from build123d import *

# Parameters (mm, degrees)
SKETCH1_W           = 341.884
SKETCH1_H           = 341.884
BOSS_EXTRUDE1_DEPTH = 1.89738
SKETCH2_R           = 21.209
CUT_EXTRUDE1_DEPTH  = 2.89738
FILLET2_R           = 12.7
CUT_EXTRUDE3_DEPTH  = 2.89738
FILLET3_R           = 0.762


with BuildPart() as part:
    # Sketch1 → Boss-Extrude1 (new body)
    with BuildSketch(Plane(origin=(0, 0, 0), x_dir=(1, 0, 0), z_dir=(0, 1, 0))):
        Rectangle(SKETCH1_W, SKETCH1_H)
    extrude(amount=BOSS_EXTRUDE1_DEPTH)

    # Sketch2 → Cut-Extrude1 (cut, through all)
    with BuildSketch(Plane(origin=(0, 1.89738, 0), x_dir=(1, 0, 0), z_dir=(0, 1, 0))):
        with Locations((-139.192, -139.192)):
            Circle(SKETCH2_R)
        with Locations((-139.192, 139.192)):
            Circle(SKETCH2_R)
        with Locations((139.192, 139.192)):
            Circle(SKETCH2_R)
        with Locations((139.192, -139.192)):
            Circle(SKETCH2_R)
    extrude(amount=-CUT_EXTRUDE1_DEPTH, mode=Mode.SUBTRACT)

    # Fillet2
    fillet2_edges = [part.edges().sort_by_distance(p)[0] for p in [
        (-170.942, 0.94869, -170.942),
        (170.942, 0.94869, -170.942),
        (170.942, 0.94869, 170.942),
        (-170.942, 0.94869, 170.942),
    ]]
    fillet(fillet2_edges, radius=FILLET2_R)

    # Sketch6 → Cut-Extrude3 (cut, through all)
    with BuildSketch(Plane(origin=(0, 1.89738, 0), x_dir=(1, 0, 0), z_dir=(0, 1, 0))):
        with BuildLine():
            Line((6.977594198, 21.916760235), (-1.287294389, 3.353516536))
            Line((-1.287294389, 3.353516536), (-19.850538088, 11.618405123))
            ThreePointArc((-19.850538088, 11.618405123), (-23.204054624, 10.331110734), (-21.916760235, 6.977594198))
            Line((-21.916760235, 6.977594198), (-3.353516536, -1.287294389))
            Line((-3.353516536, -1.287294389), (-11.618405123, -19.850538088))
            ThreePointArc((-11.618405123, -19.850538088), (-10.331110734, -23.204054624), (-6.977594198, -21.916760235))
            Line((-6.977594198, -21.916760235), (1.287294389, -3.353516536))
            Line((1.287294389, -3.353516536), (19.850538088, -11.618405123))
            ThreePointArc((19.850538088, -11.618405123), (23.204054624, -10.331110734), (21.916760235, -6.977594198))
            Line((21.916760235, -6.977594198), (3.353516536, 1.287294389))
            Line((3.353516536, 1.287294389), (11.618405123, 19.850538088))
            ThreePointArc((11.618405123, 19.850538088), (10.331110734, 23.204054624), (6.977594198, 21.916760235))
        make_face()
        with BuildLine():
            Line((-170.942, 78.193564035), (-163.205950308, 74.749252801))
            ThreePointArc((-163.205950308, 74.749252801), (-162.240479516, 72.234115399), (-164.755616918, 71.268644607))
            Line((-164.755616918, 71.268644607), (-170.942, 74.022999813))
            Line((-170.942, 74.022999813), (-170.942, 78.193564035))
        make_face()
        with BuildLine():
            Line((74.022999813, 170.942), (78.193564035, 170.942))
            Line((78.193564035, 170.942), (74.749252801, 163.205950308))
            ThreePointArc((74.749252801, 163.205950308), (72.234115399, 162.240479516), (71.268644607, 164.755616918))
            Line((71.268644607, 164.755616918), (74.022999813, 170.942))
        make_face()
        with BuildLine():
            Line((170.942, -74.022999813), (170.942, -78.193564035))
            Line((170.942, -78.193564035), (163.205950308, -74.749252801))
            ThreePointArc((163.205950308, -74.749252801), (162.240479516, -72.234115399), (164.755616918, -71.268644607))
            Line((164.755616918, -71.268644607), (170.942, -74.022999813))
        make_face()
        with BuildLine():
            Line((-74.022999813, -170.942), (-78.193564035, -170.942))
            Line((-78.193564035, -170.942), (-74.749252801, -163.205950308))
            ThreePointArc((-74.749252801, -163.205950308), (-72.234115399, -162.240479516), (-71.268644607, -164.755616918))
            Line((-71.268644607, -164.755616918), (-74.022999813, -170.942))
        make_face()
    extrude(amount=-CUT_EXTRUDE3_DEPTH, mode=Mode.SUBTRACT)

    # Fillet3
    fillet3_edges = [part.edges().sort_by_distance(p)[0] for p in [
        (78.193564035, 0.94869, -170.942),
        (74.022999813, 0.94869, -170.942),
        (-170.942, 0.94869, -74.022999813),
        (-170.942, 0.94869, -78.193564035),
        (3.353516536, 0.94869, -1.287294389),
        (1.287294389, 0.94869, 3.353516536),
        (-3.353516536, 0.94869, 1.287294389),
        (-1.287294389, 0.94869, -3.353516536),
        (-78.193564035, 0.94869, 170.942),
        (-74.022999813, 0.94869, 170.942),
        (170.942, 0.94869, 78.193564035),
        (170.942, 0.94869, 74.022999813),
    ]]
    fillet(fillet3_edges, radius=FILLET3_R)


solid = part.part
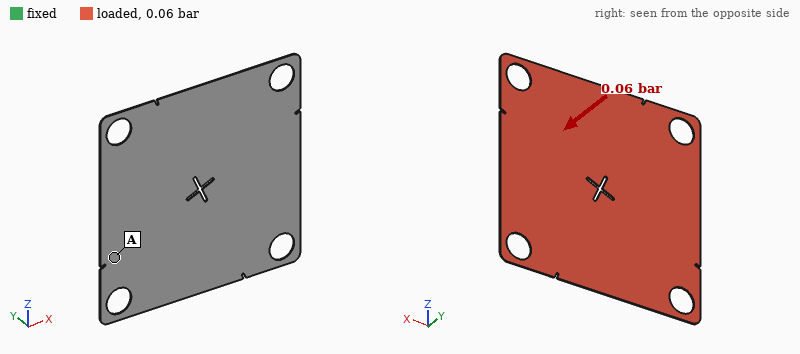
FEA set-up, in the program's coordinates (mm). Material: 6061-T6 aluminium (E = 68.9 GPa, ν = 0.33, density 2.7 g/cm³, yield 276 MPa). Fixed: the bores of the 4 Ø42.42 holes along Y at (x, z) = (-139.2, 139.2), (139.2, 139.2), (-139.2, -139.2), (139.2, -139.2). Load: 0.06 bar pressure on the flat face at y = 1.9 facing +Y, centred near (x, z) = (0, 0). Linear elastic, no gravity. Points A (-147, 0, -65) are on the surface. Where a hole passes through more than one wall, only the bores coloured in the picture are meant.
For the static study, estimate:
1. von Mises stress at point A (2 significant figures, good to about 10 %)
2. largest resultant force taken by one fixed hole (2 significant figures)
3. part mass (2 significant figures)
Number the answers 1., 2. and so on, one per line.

1. 15 MPa
2. 170 N
3. 570 g
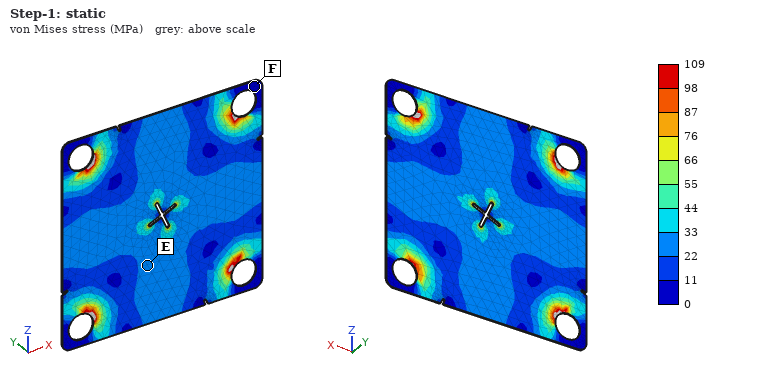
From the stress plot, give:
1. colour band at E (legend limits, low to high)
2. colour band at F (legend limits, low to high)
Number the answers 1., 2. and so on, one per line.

1. 22 to 33 MPa
2. 0 to 11 MPa
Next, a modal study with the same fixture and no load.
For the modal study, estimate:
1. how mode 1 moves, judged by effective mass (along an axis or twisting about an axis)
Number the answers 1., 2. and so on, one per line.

1. along Y
